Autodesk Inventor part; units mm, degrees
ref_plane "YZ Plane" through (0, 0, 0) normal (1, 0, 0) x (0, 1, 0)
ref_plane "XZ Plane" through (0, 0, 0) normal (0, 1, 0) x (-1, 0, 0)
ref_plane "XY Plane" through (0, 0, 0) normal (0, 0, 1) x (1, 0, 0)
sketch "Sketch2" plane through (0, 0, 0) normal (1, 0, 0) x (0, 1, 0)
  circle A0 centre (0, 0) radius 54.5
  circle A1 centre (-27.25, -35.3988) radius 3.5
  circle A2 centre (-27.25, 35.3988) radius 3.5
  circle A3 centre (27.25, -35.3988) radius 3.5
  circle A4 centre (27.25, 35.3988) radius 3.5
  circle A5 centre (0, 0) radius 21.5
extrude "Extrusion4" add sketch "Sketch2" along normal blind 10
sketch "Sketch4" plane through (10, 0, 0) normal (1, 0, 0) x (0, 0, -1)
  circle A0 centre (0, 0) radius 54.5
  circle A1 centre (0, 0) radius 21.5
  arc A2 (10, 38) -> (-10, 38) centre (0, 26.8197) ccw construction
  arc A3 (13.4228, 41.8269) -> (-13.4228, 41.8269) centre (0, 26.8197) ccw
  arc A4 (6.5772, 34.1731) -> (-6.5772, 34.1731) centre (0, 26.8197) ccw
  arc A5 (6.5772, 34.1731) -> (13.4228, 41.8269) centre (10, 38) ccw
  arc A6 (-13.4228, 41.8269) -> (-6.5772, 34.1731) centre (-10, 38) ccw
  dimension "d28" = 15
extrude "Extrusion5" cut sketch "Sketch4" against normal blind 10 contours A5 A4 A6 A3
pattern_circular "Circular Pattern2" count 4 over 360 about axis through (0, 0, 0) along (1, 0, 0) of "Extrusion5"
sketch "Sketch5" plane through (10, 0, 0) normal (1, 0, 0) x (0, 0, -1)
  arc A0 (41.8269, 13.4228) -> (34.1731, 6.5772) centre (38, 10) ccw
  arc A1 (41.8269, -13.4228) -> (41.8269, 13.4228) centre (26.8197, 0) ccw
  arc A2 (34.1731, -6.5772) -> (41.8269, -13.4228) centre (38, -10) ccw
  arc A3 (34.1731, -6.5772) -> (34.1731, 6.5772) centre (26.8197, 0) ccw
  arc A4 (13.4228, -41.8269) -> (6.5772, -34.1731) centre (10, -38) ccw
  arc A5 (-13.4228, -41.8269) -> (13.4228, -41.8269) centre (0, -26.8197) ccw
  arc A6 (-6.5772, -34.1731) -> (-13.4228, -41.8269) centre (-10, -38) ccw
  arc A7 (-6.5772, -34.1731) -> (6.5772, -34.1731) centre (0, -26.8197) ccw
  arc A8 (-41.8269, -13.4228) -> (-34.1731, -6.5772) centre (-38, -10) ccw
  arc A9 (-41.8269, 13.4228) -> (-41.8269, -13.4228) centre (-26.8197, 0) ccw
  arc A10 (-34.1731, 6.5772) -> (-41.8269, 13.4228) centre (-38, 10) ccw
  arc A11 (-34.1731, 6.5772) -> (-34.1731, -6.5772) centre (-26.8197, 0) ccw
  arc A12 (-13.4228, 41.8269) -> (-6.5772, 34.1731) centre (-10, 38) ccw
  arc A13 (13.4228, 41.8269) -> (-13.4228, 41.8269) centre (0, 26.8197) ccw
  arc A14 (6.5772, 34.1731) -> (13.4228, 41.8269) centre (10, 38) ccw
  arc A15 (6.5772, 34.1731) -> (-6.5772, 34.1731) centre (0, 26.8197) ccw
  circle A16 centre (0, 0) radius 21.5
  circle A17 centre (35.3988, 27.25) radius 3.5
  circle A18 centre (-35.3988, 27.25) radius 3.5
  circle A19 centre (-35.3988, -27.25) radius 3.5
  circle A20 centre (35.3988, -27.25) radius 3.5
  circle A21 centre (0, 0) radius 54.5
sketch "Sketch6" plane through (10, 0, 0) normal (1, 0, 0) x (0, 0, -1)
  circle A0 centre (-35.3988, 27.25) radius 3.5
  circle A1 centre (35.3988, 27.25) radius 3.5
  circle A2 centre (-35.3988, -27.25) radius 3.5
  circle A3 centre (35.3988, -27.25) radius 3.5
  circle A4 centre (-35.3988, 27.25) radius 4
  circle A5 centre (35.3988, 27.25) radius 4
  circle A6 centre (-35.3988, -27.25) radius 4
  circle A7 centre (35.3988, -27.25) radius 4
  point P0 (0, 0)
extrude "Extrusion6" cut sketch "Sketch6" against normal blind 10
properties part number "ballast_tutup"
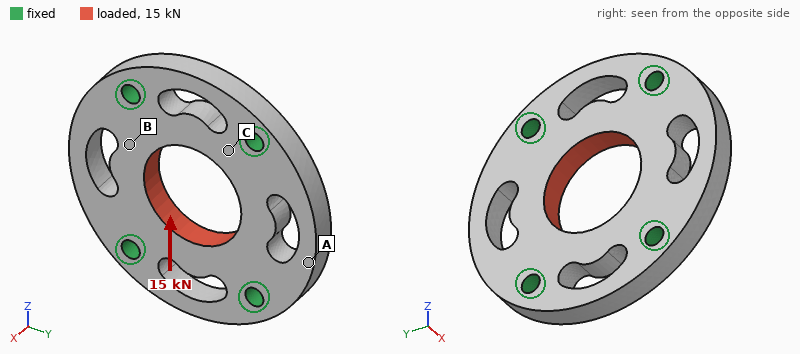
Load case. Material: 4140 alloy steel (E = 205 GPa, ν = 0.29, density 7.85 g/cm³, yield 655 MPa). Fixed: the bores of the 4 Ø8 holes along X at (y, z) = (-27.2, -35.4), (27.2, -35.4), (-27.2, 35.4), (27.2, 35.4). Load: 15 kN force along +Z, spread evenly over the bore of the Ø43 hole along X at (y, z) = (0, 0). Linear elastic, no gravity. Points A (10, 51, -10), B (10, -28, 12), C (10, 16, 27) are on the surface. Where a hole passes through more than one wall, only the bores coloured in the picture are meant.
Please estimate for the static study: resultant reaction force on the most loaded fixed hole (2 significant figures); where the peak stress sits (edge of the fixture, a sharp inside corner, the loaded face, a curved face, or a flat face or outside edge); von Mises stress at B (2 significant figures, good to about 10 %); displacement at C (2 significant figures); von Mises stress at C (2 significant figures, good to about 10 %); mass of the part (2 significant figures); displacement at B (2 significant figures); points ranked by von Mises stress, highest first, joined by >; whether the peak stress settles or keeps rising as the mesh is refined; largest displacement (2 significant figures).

3.9 kN
edge of the fixture
10 MPa
1.7 µm
18 MPa
510 g
1.5 µm
C > B > A
keeps rising
4.2 µm
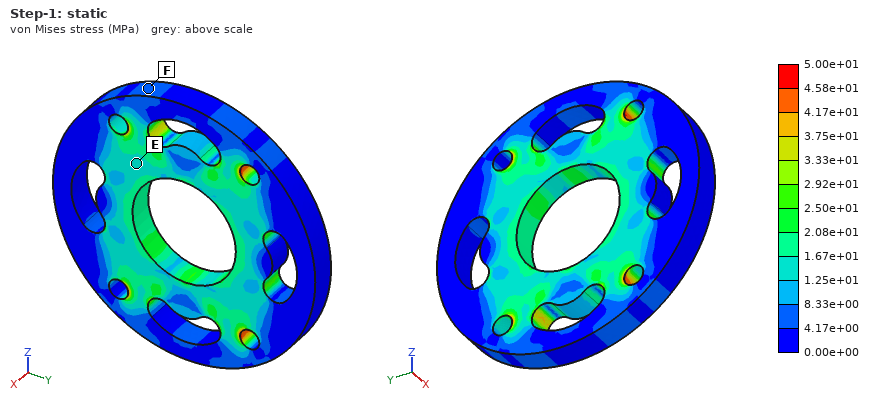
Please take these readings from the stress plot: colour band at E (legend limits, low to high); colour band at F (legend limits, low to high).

1.25e+01 to 1.67e+01 MPa
4.17e+00 to 8.33e+00 MPa
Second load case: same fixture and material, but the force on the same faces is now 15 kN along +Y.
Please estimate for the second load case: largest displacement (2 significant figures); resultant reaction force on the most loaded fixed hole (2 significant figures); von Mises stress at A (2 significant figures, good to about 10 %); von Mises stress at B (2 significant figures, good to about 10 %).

6.6 µm
3.8 kN
12 MPa
22 MPa
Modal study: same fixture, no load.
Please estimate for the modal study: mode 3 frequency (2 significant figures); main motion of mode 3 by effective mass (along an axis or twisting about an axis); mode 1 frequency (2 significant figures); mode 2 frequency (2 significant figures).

12 kHz
along X
7800 Hz
7900 Hz
